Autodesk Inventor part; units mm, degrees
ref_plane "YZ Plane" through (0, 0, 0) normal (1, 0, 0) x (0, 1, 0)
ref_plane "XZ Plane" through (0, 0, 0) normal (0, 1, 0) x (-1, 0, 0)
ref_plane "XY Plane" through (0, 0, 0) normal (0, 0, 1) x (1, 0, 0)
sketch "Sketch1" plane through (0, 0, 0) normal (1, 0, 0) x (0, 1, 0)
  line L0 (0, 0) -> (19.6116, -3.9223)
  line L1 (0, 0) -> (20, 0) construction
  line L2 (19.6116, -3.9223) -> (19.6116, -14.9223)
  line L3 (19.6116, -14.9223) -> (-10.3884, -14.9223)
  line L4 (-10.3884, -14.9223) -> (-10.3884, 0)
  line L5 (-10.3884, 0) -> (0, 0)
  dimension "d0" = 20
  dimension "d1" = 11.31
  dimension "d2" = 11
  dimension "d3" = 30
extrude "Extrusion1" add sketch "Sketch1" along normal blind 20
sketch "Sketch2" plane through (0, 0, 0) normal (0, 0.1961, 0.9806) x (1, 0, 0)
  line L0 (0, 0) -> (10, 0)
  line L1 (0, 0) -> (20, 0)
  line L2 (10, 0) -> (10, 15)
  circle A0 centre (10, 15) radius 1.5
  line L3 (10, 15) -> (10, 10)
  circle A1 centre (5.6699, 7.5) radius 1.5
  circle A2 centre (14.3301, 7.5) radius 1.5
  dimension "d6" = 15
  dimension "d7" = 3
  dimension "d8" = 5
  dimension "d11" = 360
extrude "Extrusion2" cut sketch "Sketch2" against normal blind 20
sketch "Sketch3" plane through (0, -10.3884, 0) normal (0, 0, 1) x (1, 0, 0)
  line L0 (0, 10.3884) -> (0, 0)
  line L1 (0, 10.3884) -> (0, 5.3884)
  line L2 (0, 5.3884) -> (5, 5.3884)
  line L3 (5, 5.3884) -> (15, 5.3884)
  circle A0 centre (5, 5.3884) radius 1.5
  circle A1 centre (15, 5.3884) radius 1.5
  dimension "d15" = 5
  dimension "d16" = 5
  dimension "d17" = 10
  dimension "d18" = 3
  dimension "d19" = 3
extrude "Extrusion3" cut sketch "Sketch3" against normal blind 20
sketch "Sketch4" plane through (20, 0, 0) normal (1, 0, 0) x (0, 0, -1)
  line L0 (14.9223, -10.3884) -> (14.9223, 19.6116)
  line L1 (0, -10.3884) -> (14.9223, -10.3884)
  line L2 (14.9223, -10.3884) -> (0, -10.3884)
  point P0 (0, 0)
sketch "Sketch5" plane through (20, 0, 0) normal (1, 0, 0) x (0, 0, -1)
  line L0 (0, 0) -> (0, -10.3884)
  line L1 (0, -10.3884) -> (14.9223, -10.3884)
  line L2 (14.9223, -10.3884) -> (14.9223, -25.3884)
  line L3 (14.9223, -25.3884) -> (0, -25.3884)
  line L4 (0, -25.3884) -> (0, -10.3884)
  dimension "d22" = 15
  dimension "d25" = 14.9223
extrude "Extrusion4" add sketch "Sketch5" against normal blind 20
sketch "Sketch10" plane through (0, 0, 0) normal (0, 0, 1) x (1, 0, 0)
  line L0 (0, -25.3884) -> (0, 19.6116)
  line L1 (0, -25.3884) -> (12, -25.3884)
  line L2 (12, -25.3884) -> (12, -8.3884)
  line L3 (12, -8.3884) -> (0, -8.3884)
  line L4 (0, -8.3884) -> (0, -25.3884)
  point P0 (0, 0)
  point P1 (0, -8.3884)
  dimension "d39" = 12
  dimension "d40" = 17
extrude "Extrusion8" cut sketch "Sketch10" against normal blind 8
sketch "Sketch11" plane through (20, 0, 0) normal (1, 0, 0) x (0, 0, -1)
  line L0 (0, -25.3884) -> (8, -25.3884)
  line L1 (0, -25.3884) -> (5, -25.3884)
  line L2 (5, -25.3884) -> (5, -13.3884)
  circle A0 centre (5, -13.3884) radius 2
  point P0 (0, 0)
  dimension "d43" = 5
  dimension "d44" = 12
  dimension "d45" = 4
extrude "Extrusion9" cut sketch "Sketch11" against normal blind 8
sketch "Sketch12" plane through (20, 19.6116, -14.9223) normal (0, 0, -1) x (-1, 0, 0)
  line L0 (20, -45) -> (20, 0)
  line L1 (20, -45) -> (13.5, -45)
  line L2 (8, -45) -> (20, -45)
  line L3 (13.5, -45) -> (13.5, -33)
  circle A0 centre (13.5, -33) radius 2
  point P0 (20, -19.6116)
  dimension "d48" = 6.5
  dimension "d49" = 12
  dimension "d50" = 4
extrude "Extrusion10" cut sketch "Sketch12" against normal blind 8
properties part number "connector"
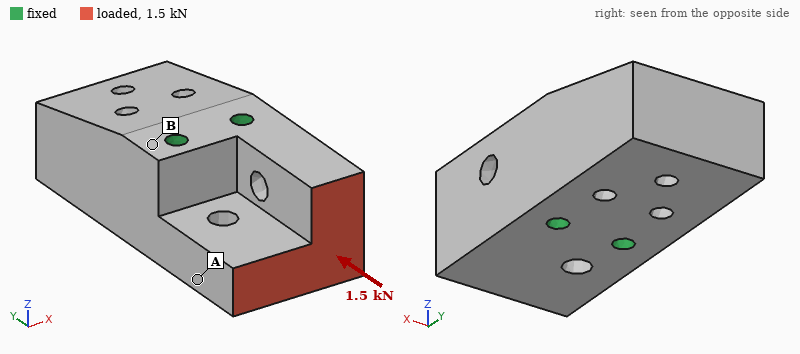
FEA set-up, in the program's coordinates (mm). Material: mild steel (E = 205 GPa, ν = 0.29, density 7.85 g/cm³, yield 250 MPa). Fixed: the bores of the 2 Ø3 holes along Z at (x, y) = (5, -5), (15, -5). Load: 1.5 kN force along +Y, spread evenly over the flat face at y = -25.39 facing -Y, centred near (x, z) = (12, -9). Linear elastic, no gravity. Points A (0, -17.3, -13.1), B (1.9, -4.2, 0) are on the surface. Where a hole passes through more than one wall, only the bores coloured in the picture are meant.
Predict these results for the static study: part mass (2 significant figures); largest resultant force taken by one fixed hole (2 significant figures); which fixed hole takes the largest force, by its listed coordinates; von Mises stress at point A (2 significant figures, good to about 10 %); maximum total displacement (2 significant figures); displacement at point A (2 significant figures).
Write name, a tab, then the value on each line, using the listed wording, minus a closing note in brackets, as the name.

part mass	81 g
largest resultant force taken by one fixed hole	1.0 kN
which fixed hole takes the largest force, by its listed coordinates	(15, -5)
von Mises stress at point A	8.4 MPa
maximum total displacement	0.92 µm
displacement at point A	0.52 µm
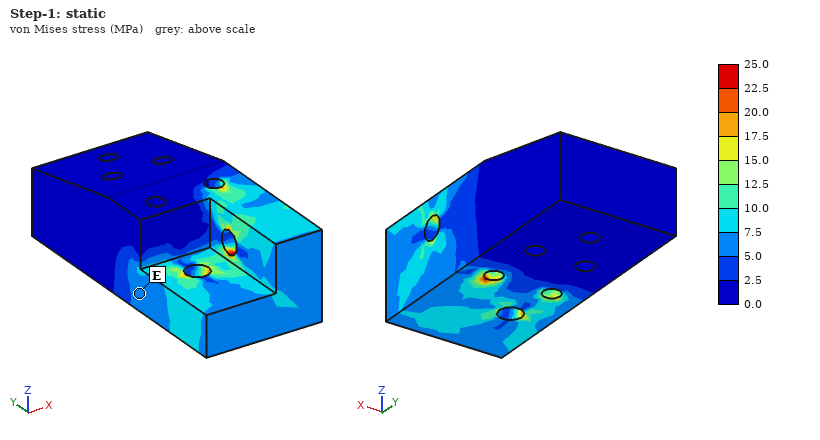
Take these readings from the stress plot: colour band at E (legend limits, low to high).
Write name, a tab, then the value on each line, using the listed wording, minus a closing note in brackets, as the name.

colour band at E	5.0 to 7.5 MPa
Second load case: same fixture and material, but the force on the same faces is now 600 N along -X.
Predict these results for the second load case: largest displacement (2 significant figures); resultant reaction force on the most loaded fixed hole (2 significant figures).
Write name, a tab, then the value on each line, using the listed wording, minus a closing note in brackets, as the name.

largest displacement	4.5 µm
resultant reaction force on the most loaded fixed hole	1.0 kN
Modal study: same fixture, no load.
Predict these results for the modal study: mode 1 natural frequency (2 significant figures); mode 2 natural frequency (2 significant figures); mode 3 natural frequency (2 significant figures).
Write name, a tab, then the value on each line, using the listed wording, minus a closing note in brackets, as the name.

mode 1 natural frequency	17 kHz
mode 2 natural frequency	18 kHz
mode 3 natural frequency	19 kHz
